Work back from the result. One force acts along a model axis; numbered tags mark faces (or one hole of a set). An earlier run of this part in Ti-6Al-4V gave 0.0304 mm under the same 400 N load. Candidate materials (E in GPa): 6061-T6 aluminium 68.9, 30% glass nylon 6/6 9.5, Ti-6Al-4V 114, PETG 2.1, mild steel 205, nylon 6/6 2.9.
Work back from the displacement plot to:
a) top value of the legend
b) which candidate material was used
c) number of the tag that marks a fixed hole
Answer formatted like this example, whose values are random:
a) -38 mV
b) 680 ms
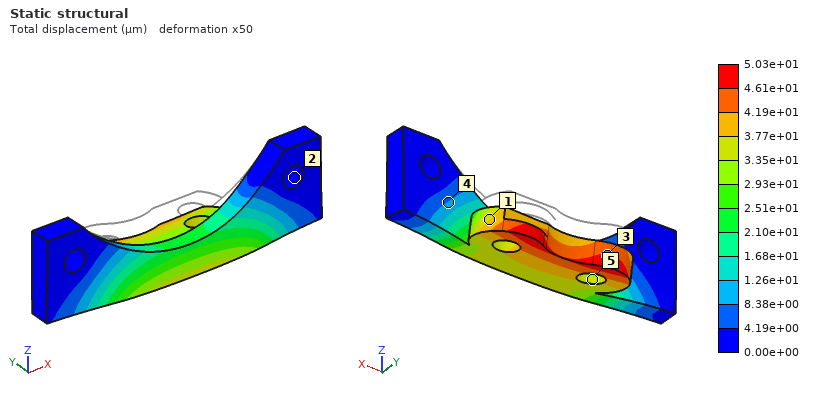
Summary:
a) 5.03e+01 µm
b) 6061-T6 aluminium
c) 2
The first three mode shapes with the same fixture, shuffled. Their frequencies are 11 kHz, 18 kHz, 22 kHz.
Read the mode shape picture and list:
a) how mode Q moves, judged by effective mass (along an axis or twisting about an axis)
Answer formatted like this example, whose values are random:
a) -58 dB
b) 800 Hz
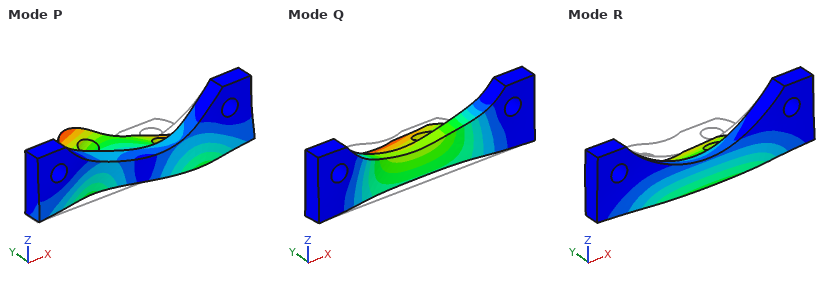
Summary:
a) along Y
